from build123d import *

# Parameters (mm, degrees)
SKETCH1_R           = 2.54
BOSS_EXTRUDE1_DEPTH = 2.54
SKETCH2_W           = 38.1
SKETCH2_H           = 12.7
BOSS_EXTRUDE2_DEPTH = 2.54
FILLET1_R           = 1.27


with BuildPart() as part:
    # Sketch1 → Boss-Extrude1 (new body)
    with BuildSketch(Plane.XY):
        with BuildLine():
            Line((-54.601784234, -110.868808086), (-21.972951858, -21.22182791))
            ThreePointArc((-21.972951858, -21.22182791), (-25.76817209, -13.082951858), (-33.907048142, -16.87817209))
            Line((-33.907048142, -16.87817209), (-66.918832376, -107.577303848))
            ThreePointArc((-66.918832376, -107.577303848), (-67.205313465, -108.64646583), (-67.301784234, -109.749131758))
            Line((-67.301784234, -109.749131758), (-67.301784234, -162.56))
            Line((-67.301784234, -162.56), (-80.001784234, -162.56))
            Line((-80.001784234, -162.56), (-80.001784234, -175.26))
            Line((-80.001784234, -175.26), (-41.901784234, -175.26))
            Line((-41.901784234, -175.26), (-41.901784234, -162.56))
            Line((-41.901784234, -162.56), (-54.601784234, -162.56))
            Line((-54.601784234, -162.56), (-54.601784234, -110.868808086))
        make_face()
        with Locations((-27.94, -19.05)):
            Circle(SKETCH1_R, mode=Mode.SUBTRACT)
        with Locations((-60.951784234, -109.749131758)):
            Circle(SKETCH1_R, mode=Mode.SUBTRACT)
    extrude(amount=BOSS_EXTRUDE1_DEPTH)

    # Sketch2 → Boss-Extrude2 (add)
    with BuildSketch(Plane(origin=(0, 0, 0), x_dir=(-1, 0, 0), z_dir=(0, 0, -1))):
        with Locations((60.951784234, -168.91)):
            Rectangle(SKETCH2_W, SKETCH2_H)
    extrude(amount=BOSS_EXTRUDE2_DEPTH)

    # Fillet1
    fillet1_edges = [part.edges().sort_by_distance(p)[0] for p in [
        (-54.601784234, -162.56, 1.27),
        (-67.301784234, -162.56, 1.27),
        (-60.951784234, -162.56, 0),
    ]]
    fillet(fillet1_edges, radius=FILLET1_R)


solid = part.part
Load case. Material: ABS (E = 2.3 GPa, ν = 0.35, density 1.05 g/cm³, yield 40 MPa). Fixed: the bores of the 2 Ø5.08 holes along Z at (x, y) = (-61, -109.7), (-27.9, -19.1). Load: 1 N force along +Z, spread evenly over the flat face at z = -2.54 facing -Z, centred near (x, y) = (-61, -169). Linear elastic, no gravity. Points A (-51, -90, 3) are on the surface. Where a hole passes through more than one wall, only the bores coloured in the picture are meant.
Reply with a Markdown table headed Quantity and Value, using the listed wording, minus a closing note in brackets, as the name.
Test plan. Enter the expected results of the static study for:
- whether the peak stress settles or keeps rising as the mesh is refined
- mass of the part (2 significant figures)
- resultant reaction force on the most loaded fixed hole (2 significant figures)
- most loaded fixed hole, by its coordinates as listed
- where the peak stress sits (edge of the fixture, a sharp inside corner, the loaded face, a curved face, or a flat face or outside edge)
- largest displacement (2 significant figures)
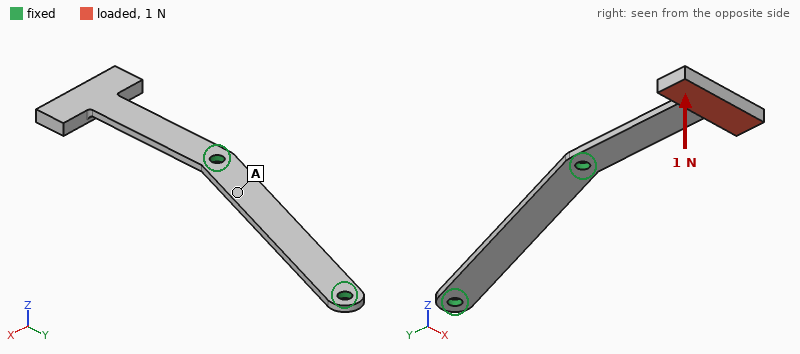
| Quantity | Value |
|---|---|
| whether the peak stress settles or keeps rising as the mesh is refined | keeps rising |
| mass of the part | 7.7 g |
| resultant reaction force on the most loaded fixed hole | 1.00 N |
| most loaded fixed hole, by its coordinates as listed | (-61, -109.7) |
| where the peak stress sits | edge of the fixture |
| largest displacement | 1.8 mm |
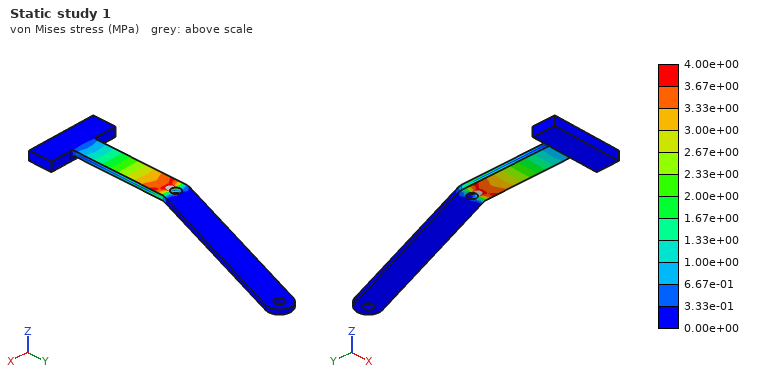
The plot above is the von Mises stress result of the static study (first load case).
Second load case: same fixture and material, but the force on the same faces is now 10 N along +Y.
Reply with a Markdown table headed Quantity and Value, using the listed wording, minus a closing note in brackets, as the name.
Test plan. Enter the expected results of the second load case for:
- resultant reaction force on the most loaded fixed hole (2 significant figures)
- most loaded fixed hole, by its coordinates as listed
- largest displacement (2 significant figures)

| Quantity | Value |
|---|---|
| resultant reaction force on the most loaded fixed hole | 9.9 N |
| most loaded fixed hole, by its coordinates as listed | (-61, -109.7) |
| largest displacement | 1.9 mm |
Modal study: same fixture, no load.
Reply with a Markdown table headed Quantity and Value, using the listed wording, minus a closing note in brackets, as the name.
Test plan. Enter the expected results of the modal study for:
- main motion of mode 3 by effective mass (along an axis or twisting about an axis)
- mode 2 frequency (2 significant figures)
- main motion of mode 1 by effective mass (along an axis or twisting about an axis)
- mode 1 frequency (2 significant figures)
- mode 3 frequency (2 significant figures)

| Quantity | Value |
|---|---|
| main motion of mode 3 by effective mass | along X |
| mode 2 frequency | 280 Hz |
| main motion of mode 1 by effective mass | along Z |
| mode 1 frequency | 75 Hz |
| mode 3 frequency | 320 Hz |
